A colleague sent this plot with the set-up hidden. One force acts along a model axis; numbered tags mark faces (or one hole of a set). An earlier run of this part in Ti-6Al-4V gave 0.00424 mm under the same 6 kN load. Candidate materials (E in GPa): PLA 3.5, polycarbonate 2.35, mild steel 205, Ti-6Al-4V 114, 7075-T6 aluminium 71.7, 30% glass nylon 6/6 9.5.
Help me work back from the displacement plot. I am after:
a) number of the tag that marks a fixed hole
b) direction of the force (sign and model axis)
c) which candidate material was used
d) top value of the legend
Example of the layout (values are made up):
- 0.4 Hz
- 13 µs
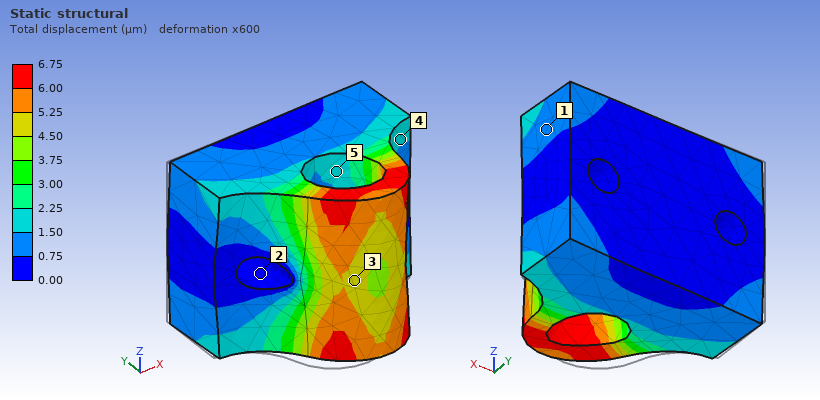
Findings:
- 2
- +X
- 7075-T6 aluminium
- 6.75 µm
